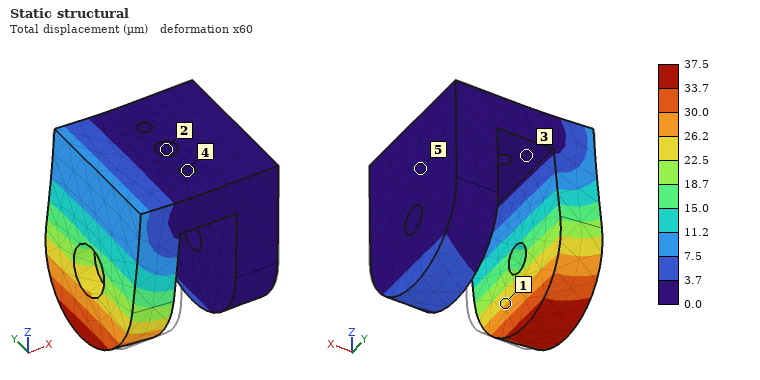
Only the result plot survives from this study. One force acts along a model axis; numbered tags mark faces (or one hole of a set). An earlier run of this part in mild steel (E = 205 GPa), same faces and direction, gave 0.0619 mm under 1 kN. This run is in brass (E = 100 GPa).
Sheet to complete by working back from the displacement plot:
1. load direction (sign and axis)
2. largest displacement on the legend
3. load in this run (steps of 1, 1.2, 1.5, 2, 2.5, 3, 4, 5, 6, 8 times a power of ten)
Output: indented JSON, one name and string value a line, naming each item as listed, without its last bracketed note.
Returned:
{
  "load direction": "-X",
  "largest displacement on the legend": "37.5 µm",
  "load in this run": "300 N"
}
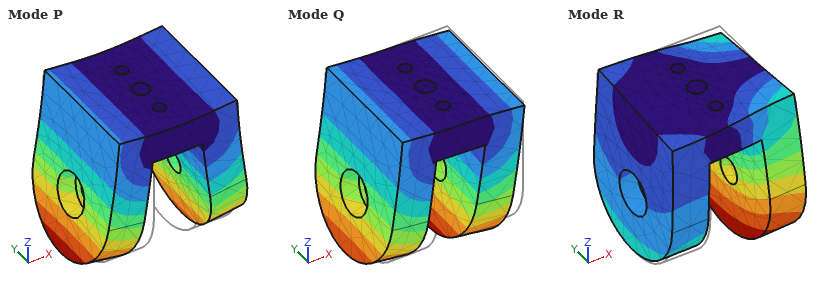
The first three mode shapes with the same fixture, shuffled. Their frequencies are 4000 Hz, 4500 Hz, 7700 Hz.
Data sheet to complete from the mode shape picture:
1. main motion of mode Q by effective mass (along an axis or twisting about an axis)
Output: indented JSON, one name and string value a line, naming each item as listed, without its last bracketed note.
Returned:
{
  "main motion of mode Q by effective mass": "along X"
}
